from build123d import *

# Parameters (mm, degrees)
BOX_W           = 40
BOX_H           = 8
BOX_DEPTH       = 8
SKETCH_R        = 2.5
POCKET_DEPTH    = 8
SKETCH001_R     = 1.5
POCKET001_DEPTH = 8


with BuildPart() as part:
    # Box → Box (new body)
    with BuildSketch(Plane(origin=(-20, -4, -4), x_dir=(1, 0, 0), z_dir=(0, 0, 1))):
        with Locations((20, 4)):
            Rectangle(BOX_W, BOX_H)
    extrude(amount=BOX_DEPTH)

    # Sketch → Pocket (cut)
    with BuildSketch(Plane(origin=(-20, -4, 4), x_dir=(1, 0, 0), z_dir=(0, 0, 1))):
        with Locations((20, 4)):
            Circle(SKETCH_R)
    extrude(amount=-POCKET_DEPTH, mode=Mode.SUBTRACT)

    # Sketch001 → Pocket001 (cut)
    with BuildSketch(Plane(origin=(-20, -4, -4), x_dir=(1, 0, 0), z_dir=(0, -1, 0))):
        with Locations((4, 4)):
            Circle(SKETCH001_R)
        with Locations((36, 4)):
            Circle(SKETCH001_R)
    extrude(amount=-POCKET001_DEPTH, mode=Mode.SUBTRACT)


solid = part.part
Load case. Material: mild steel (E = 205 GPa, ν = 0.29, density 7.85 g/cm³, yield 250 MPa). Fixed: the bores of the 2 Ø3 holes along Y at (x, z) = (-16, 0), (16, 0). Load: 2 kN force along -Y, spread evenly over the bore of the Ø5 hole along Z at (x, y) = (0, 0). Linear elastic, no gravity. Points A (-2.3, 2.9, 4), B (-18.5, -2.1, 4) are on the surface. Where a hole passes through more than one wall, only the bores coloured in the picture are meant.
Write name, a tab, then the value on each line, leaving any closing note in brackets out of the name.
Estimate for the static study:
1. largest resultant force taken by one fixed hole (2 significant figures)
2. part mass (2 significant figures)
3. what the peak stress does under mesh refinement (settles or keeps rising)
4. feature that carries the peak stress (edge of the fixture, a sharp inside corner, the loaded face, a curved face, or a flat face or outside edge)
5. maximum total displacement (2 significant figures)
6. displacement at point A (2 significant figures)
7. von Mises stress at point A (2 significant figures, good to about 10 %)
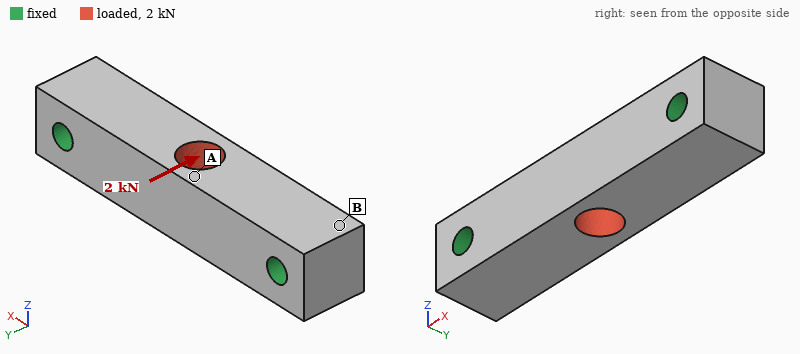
largest resultant force taken by one fixed hole	1.0 kN
part mass	18 g
what the peak stress does under mesh refinement	keeps rising
feature that carries the peak stress	edge of the fixture
maximum total displacement	8.2 µm
displacement at point A	7.5 µm
von Mises stress at point A	52 MPa
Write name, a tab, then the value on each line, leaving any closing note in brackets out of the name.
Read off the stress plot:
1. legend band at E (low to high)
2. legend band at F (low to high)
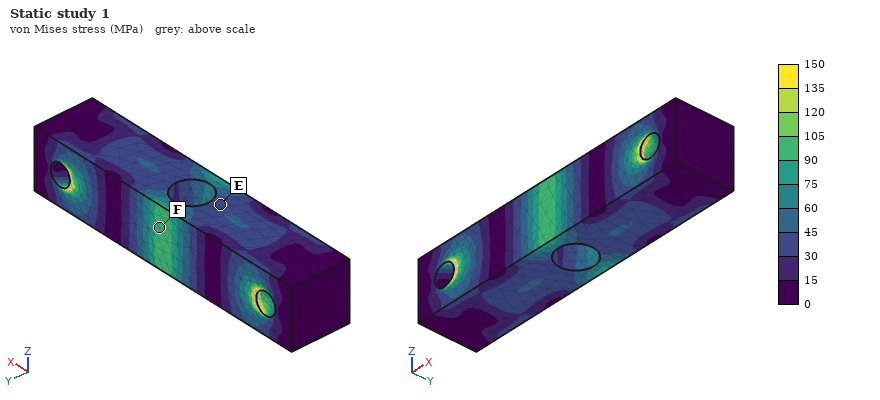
legend band at E	30 to 45 MPa
legend band at F	90 to 105 MPa
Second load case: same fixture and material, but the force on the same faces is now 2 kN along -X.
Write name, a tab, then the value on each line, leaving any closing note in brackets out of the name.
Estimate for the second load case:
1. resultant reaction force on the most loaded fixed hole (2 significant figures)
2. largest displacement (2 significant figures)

resultant reaction force on the most loaded fixed hole	1.0 kN
largest displacement	1.2 µm
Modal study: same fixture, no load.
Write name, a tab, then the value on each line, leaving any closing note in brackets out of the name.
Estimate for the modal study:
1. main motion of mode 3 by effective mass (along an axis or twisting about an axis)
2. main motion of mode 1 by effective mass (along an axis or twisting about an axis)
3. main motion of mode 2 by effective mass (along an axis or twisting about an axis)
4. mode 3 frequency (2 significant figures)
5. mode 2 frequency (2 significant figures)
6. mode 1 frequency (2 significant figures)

main motion of mode 3 by effective mass	twisting about X
main motion of mode 1 by effective mass	along Z
main motion of mode 2 by effective mass	along Y
mode 3 frequency	50 kHz
mode 2 frequency	35 kHz
mode 1 frequency	27 kHz
